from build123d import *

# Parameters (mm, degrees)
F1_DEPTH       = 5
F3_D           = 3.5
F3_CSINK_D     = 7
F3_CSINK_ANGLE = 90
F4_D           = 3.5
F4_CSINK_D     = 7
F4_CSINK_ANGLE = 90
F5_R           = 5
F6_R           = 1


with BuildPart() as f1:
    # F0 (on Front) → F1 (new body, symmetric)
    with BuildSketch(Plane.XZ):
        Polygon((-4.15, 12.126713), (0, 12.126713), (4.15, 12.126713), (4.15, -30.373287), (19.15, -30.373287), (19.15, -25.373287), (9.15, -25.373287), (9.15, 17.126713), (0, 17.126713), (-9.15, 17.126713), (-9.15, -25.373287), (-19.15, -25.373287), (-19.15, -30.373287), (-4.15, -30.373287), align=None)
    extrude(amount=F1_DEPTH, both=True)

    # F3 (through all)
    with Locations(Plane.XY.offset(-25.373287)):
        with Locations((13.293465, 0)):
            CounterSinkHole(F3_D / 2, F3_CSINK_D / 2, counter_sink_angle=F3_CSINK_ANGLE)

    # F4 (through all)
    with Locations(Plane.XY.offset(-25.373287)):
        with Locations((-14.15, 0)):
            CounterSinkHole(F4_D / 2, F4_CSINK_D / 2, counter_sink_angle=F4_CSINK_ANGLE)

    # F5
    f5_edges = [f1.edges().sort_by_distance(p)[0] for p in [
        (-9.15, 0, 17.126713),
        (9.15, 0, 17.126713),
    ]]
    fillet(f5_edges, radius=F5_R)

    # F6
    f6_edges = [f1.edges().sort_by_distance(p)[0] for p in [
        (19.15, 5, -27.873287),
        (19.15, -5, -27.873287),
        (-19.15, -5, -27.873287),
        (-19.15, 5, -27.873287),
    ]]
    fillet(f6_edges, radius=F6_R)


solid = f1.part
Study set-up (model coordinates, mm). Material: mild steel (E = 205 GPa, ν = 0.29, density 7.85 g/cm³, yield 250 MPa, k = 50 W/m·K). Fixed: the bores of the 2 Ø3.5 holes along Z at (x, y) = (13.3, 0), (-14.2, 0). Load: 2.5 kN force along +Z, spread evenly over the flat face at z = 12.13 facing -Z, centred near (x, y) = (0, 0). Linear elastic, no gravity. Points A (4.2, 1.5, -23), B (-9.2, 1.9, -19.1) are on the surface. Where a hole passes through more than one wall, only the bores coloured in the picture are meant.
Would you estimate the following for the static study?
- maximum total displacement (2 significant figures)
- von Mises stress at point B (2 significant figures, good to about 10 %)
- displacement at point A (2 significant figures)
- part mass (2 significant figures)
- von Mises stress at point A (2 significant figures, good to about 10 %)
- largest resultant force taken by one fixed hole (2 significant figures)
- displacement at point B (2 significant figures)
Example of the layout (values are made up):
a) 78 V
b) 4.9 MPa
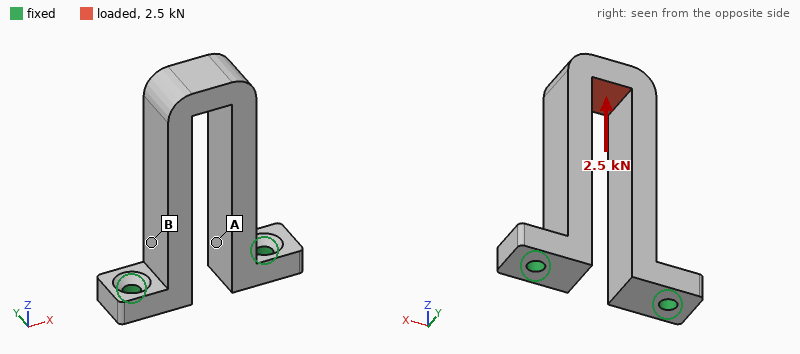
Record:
a) 16 µm
b) 72 MPa
c) 9.1 µm
d) 46 g
e) 26 MPa
f) 1.3 kN
g) 11 µm
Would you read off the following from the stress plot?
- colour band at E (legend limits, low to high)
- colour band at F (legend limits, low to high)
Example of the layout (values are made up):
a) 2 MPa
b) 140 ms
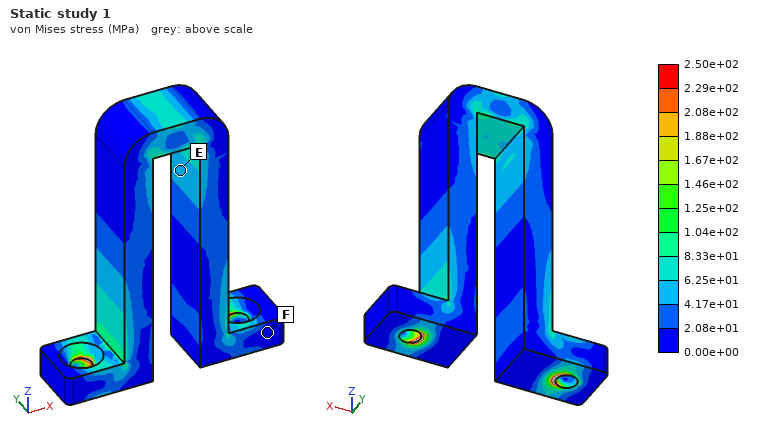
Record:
a) 4.17e+01 to 6.25e+01 MPa
b) 0.00e+00 to 2.08e+01 MPa
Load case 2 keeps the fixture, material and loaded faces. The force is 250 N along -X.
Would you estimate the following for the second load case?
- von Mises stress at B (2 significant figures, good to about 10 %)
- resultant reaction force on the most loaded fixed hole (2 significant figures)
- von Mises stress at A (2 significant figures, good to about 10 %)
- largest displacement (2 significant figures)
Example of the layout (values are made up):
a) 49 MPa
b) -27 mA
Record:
a) 43 MPa
b) 380 N
c) 39 MPa
d) 48 µm
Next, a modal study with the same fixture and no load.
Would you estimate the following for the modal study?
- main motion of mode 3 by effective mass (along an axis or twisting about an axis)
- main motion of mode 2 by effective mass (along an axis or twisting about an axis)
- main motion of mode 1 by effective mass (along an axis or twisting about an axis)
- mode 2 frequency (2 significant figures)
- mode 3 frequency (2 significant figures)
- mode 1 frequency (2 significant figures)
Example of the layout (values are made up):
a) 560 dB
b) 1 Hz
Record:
a) twisting about Z
b) along X
c) along Y
d) 2800 Hz
e) 6500 Hz
f) 2000 Hz
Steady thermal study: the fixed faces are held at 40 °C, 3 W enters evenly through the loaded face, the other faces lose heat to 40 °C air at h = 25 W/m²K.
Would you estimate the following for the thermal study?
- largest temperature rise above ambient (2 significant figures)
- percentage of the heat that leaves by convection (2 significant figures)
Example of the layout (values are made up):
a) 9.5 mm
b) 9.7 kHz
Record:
a) 25 K
b) 30 %
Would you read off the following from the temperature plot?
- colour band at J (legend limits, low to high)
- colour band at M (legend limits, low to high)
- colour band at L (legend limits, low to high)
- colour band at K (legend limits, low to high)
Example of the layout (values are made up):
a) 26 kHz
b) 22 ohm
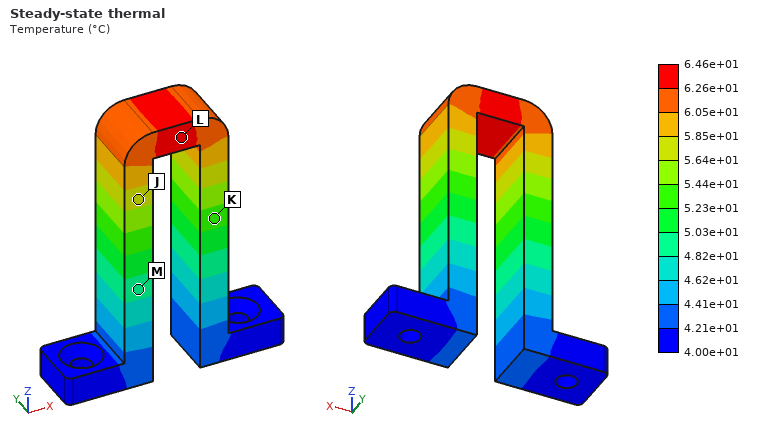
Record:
a) 5.64e+01 to 5.85e+01 °C
b) 4.82e+01 to 5.03e+01 °C
c) 6.26e+01 to 6.46e+01 °C
d) 5.23e+01 to 5.44e+01 °C
